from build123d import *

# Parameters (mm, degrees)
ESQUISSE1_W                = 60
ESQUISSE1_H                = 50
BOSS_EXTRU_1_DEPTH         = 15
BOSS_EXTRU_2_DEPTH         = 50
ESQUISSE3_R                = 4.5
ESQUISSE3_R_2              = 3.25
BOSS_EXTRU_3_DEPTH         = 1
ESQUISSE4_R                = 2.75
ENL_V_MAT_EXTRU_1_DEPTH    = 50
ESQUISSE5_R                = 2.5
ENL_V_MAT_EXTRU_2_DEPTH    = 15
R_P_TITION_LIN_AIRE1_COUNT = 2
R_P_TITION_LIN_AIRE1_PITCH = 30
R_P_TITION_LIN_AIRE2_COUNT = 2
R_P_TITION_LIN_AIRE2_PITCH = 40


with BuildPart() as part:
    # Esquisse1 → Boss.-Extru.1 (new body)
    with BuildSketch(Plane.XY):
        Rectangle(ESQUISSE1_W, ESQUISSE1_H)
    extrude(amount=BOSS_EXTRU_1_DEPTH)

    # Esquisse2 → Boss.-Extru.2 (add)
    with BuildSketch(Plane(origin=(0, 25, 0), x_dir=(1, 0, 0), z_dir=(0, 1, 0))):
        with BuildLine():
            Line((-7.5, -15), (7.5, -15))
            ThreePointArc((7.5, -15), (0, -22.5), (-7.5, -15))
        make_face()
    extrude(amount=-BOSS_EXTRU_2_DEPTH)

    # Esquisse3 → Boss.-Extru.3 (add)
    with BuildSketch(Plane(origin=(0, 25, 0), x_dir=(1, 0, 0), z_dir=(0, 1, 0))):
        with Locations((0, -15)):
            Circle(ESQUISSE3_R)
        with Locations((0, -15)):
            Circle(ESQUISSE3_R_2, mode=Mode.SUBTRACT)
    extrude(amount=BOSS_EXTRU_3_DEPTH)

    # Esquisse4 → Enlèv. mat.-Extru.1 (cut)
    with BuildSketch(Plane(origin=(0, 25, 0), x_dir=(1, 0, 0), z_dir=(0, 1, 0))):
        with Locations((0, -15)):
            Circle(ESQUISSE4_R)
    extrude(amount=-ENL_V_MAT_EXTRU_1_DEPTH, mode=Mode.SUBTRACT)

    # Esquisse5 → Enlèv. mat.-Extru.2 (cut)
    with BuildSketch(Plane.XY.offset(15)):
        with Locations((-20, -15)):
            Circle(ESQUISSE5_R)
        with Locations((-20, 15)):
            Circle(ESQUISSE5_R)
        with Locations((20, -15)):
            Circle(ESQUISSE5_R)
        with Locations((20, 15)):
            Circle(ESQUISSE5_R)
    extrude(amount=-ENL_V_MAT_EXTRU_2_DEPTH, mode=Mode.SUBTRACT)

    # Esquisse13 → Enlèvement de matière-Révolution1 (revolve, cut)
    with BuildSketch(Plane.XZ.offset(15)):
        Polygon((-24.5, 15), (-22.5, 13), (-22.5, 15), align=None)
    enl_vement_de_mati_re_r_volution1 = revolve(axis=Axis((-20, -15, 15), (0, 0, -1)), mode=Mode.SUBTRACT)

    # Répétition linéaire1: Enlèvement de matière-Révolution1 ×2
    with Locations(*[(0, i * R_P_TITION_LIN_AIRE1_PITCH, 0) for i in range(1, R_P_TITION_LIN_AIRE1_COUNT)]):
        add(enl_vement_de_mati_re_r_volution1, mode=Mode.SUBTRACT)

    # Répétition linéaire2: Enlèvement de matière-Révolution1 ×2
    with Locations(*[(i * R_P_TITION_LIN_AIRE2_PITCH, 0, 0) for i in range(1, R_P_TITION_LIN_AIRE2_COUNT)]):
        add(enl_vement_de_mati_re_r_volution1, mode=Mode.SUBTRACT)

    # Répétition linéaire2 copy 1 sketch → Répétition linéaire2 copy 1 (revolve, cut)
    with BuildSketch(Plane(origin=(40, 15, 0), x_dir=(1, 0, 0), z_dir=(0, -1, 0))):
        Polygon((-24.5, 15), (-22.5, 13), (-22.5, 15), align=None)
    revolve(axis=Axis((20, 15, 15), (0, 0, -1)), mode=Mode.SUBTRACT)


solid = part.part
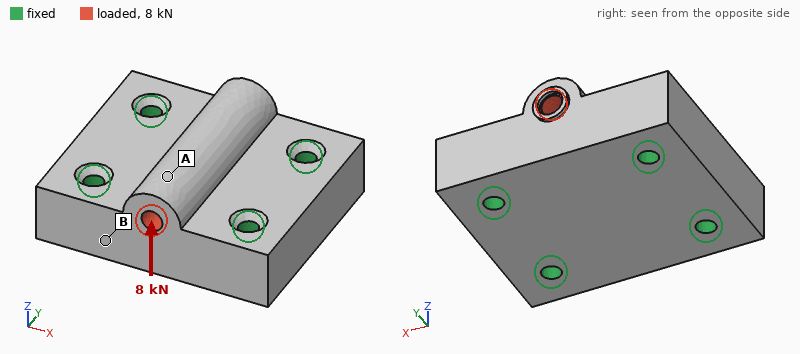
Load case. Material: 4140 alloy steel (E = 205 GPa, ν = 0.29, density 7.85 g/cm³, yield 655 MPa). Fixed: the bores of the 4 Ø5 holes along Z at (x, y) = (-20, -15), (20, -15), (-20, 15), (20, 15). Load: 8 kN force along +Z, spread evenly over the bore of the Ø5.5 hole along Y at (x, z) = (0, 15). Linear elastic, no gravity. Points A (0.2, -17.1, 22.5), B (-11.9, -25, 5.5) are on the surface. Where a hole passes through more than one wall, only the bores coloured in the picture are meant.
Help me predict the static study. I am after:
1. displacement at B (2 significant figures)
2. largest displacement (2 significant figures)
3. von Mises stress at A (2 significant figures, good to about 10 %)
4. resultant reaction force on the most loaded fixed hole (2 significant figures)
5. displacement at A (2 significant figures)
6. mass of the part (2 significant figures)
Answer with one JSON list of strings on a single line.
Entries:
["1.3 µm", "2.7 µm", "5.3 MPa", "2.0 kN", "2.4 µm", "370 g"]
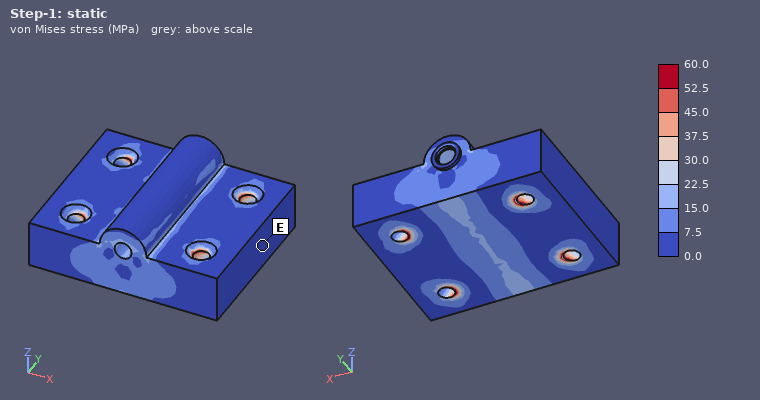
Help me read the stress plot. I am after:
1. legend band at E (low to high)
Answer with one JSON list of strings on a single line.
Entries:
["0.0 to 7.5 MPa"]
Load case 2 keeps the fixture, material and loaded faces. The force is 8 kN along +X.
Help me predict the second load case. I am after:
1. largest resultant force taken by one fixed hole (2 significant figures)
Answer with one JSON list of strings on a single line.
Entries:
["2.2 kN"]
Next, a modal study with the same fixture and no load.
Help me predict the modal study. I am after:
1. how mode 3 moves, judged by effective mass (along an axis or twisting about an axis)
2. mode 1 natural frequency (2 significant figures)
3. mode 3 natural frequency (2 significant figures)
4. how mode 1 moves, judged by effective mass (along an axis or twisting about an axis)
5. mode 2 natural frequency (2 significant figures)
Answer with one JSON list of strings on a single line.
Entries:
["along Y", "23 kHz", "32 kHz", "along Z", "26 kHz"]
